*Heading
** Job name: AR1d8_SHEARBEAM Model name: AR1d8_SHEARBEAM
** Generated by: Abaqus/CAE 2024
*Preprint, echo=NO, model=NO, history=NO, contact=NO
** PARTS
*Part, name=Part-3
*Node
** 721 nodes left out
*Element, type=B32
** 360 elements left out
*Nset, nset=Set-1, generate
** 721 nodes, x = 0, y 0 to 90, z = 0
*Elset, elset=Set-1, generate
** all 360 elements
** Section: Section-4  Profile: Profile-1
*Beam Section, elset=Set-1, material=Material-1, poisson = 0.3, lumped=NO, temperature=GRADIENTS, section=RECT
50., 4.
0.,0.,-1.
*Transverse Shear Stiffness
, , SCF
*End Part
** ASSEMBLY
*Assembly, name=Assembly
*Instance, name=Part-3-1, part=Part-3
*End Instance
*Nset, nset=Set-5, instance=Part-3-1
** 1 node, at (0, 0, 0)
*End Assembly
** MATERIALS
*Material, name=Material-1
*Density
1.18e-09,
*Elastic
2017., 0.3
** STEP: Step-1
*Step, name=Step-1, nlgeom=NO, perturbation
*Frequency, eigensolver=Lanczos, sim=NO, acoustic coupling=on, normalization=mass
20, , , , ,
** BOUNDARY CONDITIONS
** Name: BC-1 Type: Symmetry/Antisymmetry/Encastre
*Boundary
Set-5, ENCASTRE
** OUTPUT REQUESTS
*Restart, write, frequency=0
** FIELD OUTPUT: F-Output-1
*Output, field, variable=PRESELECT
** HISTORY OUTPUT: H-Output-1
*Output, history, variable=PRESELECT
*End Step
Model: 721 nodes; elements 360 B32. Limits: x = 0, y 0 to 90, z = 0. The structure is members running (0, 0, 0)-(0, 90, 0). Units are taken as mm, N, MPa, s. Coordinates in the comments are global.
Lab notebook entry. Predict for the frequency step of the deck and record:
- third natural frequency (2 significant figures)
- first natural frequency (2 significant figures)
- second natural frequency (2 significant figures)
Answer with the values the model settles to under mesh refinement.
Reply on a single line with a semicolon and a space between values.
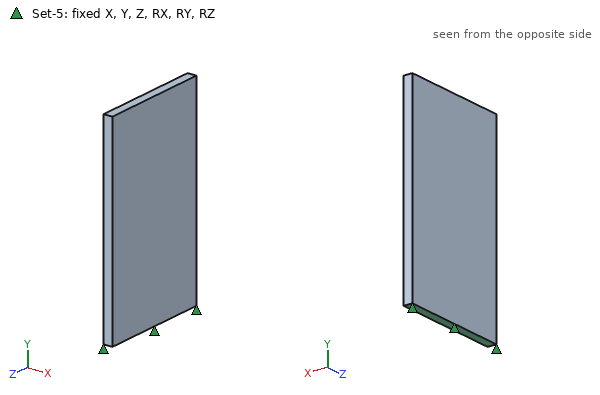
660 Hz; 110 Hz; 360 Hz
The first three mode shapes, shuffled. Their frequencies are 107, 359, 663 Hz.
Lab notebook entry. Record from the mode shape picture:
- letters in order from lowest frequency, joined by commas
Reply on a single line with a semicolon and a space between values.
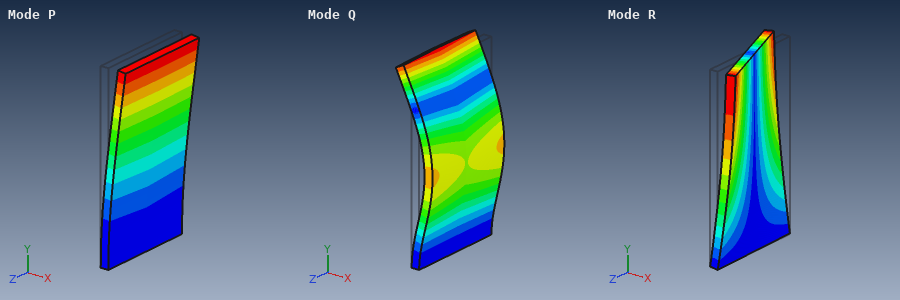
P, R, Q
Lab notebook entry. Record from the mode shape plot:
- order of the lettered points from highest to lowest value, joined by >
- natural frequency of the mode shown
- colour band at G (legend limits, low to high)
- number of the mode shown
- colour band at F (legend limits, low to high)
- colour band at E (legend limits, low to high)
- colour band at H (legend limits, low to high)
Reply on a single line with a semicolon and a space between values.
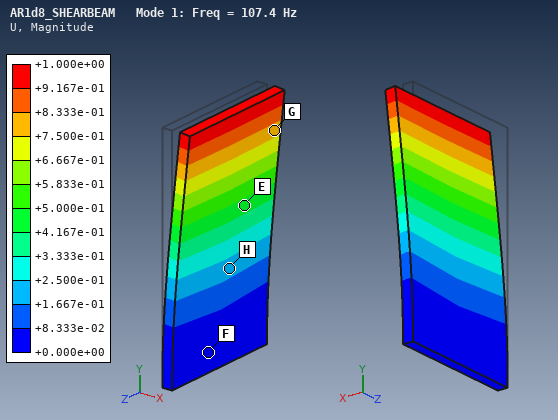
G > E > H > F; 107.4 Hz; +7.500e-01 to +8.333e-01; 1; +0.000e+00 to +8.333e-02; +4.167e-01 to +5.000e-01; +1.667e-01 to +2.500e-01
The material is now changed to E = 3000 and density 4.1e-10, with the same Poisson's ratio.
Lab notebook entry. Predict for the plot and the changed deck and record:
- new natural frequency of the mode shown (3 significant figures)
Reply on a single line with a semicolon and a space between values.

222 Hz
